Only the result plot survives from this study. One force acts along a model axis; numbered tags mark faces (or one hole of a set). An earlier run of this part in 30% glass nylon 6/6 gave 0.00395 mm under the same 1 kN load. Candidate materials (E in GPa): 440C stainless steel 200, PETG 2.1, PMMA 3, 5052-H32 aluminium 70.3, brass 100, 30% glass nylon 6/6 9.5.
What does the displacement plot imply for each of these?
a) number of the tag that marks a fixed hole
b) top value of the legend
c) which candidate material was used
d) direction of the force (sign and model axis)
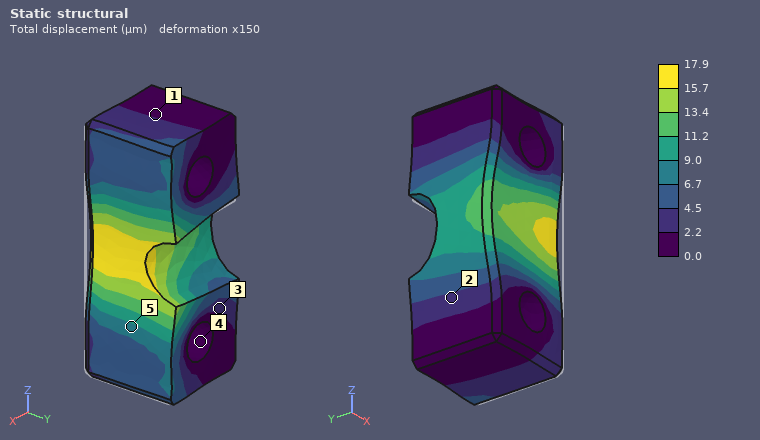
4
17.9 µm
PETG
-X
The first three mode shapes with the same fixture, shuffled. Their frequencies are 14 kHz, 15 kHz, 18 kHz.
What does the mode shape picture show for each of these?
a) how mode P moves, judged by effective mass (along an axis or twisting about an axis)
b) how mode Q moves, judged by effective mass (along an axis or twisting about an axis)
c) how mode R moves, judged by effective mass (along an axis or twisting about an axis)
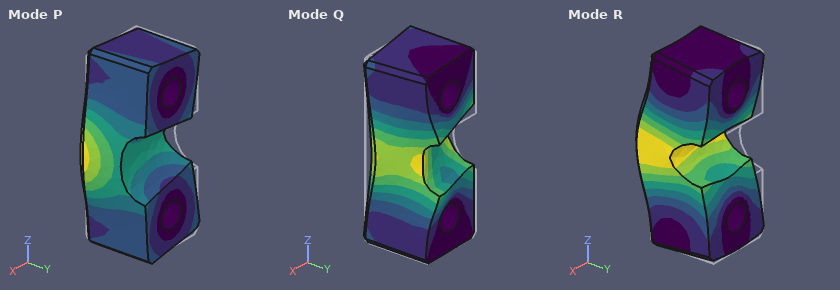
along X
twisting about Z
along Y
